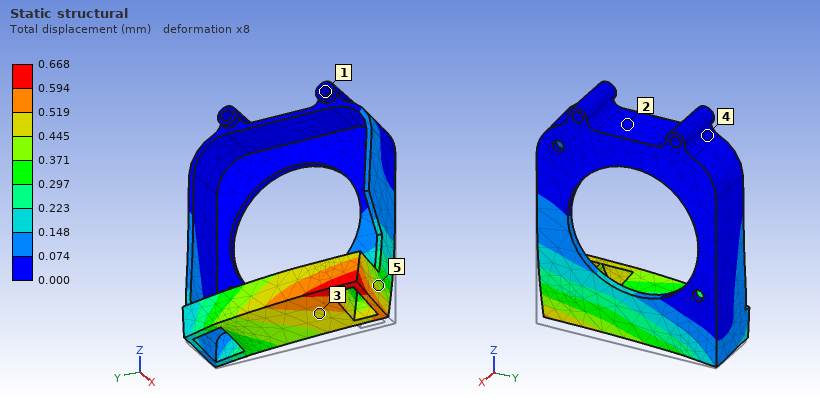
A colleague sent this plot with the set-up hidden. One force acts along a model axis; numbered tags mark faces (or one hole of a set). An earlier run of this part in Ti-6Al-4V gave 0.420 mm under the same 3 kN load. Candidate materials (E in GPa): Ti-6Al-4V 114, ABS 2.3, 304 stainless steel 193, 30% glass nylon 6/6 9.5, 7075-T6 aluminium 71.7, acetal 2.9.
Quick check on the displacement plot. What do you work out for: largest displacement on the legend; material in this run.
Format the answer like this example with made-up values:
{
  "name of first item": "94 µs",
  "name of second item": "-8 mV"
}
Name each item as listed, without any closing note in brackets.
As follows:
{
  "largest displacement on the legend": "0.668 mm",
  "material in this run": "7075-T6 aluminium"
}
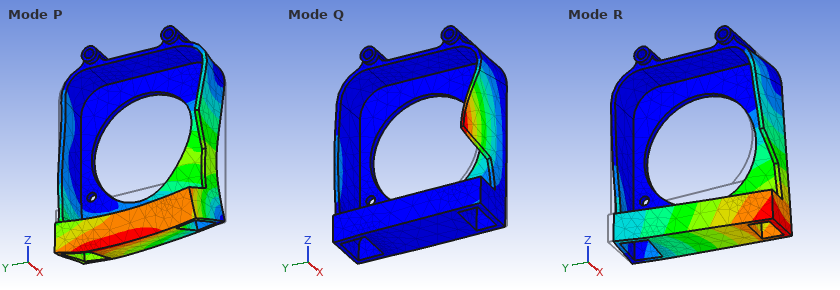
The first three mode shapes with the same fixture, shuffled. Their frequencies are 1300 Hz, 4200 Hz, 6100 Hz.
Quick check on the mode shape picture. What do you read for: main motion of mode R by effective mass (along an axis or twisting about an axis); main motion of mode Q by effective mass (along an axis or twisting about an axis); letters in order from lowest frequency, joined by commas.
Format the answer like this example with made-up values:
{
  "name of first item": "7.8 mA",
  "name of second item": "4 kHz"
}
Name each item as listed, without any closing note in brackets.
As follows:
{
  "main motion of mode R by effective mass": "along X",
  "main motion of mode Q by effective mass": "along Y",
  "letters in order from lowest frequency, joined by commas": "R, P, Q"
}
